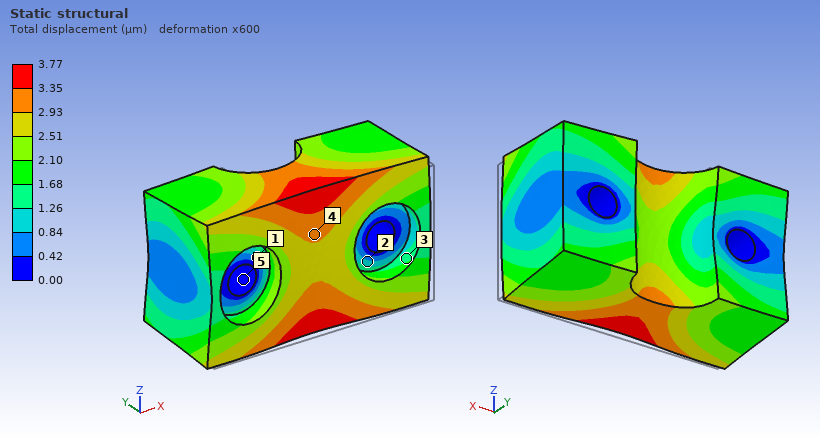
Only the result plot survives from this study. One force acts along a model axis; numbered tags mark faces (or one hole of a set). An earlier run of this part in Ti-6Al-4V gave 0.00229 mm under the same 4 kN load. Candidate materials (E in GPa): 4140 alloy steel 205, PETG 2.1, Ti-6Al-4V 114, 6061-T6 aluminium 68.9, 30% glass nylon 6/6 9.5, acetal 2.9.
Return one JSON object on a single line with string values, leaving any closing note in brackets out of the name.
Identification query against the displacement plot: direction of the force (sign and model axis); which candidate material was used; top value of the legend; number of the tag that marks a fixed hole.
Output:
{"direction of the force": "+Y", "which candidate material was used": "6061-T6 aluminium", "top value of the legend": "3.77 µm", "number of the tag that marks a fixed hole": "5"}
